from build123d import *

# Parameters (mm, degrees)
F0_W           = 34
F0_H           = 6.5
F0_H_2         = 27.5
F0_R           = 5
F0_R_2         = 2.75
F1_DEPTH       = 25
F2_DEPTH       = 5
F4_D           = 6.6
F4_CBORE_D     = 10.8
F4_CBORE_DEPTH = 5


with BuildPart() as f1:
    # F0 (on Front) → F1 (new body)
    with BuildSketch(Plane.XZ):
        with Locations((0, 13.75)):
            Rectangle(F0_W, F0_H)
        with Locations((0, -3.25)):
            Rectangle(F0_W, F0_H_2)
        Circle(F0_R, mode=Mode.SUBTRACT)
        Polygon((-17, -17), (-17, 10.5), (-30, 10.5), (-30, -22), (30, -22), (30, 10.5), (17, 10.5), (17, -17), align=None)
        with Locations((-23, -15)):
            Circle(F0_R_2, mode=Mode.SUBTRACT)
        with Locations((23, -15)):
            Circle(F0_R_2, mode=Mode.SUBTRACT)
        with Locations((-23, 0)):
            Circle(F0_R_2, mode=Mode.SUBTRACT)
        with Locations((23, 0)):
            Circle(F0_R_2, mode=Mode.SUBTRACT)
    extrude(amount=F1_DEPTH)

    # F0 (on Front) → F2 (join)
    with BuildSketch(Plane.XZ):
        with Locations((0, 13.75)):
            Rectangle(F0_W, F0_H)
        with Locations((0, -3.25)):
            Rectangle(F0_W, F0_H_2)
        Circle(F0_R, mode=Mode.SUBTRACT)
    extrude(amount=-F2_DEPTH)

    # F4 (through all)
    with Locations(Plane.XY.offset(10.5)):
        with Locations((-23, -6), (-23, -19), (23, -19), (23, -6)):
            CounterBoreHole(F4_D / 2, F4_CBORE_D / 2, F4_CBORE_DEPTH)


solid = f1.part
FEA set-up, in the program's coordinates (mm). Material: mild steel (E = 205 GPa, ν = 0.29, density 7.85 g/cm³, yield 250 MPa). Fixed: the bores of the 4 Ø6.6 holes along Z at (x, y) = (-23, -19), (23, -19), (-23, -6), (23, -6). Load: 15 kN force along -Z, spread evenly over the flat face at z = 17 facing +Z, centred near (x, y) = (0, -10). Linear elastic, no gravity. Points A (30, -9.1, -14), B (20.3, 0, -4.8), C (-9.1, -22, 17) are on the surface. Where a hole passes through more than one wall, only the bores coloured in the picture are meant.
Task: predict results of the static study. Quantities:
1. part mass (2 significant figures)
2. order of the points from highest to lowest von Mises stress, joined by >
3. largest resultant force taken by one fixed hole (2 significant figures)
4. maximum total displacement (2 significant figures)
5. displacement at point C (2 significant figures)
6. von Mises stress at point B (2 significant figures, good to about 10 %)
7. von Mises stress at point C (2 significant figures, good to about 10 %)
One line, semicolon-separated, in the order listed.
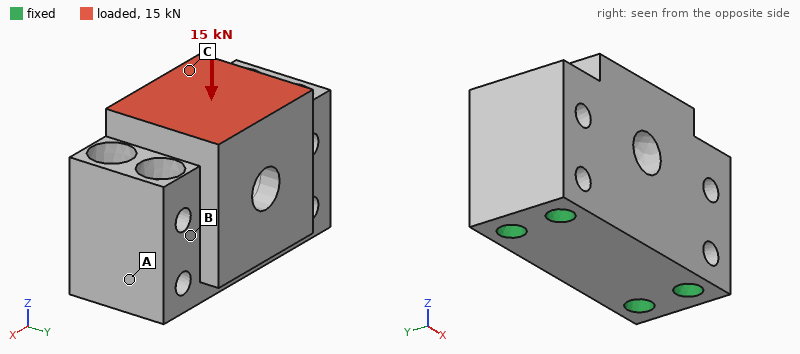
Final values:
400 g; B > C > A; 4.6 kN; 4.0 µm; 2.4 µm; 20 MPa; 13 MPa
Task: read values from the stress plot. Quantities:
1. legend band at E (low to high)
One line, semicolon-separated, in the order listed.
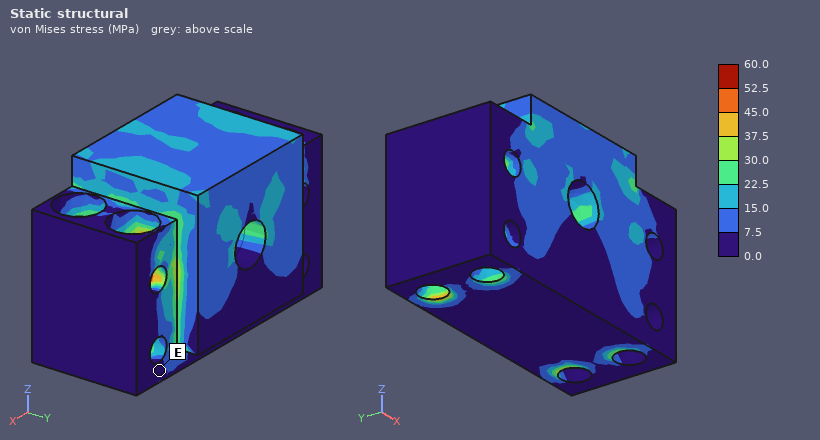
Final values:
0.0 to 7.5 MPa
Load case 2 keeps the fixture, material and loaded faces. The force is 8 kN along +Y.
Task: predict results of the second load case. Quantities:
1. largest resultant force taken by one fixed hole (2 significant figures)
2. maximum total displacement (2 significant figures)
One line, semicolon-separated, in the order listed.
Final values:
4.1 kN; 8.7 µm
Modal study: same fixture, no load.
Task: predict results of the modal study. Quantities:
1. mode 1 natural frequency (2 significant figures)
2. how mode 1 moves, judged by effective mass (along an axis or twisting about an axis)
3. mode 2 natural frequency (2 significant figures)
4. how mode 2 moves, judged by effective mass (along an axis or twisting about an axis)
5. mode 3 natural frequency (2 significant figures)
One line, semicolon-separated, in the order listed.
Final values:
20 kHz; along Y; 29 kHz; along Z; 31 kHz
